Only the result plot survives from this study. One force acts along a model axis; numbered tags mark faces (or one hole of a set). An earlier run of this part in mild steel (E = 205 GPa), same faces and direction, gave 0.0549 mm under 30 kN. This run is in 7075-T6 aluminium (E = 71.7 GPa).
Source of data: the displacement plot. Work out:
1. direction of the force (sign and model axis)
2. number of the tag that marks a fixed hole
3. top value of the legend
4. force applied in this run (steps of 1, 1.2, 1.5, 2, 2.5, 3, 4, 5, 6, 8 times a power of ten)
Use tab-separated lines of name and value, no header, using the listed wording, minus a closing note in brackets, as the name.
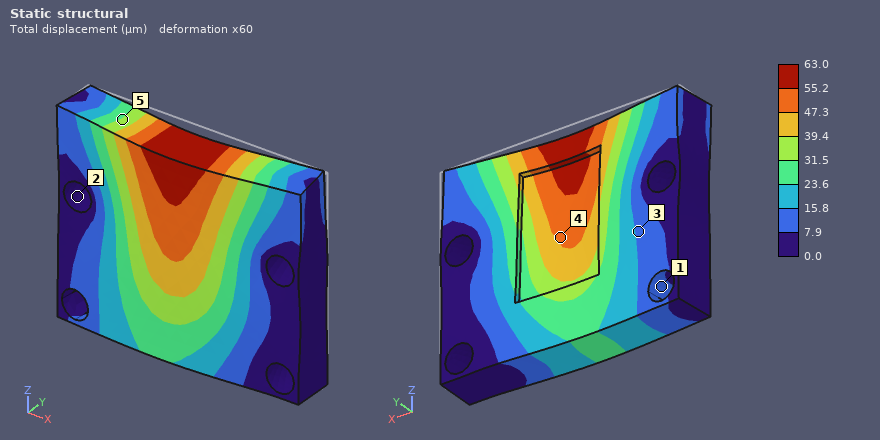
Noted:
direction of the force	-Y
number of the tag that marks a fixed hole	2
top value of the legend	63.0 µm
force applied in this run	12 kN
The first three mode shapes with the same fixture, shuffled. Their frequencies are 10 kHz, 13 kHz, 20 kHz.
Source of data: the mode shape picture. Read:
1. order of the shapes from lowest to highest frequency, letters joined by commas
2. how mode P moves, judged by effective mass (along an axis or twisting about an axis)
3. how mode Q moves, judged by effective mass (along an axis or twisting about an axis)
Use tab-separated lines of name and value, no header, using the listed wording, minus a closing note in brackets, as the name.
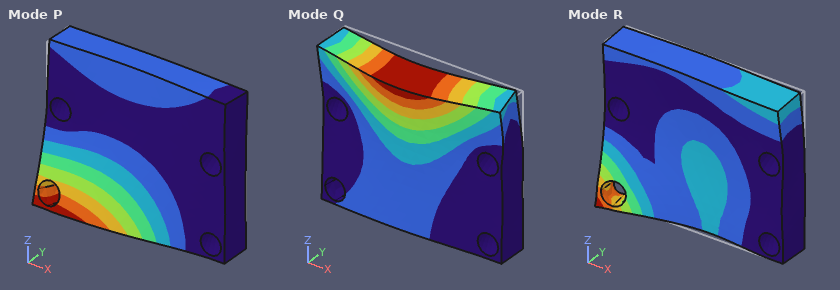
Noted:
order of the shapes from lowest to highest frequency, letters joined by commas	P, Q, R
how mode P moves, judged by effective mass	along Y
how mode Q moves, judged by effective mass	along Y
